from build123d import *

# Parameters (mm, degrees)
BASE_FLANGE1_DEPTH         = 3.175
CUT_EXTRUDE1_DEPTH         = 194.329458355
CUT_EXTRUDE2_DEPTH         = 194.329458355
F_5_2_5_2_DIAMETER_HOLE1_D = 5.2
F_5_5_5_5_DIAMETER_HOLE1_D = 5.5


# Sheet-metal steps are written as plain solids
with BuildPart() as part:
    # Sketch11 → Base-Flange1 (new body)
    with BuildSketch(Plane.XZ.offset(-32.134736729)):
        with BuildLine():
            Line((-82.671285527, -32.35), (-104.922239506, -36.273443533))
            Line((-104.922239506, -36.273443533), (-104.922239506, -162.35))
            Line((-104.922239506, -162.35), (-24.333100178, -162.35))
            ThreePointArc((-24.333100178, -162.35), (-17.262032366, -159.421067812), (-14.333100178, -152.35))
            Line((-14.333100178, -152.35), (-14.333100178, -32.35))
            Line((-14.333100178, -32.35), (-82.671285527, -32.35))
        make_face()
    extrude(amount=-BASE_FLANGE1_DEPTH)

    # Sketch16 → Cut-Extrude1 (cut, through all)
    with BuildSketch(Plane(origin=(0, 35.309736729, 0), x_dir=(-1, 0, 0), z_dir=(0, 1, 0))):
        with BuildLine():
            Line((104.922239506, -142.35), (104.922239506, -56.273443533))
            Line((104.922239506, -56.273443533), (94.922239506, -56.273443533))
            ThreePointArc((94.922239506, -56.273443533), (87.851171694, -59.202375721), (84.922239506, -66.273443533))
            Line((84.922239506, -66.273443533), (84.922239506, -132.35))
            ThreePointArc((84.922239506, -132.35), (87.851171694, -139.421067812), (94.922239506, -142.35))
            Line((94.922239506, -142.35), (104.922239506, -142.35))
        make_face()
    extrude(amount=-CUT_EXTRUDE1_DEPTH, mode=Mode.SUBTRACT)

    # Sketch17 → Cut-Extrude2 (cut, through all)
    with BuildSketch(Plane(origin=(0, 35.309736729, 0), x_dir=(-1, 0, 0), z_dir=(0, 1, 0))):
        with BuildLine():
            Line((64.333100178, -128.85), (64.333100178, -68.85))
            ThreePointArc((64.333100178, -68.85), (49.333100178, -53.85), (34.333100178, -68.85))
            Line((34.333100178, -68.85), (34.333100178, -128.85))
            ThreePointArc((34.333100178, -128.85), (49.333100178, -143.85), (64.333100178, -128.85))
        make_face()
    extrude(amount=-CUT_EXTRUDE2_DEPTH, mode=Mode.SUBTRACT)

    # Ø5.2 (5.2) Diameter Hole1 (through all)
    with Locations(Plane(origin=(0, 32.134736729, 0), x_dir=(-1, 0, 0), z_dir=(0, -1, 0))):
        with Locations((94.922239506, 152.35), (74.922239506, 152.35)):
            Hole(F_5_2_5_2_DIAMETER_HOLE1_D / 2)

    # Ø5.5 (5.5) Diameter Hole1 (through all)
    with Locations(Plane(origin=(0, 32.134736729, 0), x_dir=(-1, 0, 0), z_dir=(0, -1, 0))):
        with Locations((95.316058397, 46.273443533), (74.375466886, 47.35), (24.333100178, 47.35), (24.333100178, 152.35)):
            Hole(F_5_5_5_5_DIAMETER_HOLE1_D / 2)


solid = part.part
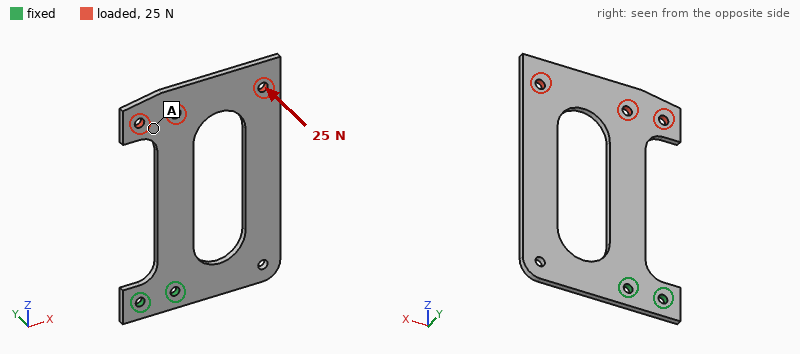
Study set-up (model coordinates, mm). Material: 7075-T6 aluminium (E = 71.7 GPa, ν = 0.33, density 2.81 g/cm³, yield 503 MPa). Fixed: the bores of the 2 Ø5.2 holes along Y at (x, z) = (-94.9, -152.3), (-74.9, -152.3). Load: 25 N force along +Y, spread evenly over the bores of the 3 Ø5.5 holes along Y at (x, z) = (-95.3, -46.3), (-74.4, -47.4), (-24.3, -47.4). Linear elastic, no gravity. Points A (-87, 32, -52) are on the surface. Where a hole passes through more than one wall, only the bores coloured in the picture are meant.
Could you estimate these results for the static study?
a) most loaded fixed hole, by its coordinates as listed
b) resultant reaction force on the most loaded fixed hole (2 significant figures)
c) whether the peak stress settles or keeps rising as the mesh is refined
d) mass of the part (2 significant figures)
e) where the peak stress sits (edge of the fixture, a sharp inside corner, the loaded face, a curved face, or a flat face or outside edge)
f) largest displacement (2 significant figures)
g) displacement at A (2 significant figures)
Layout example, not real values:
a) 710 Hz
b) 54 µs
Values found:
a) (-74.9, -152.3)
b) 38 N
c) keeps rising
d) 66 g
e) edge of the fixture
f) 1.8 mm
g) 1.3 mm
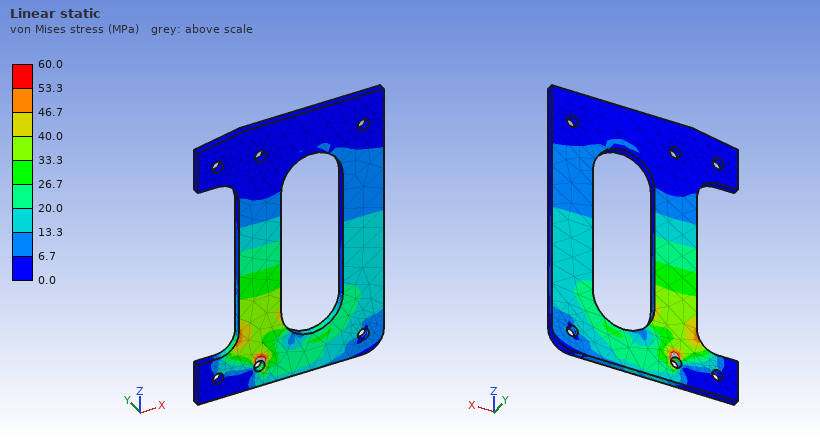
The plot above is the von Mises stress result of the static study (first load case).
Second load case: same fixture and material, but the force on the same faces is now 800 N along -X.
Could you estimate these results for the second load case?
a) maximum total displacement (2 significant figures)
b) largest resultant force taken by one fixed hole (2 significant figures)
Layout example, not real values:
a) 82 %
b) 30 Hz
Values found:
a) 0.94 mm
b) 3.6 kN
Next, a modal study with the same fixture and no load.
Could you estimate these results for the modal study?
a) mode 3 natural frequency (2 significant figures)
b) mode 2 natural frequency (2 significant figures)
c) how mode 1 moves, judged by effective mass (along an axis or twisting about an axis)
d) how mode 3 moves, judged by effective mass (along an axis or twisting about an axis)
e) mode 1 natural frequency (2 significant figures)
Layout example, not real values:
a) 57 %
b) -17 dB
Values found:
a) 720 Hz
b) 320 Hz
c) along Y
d) along Y
e) 130 Hz
